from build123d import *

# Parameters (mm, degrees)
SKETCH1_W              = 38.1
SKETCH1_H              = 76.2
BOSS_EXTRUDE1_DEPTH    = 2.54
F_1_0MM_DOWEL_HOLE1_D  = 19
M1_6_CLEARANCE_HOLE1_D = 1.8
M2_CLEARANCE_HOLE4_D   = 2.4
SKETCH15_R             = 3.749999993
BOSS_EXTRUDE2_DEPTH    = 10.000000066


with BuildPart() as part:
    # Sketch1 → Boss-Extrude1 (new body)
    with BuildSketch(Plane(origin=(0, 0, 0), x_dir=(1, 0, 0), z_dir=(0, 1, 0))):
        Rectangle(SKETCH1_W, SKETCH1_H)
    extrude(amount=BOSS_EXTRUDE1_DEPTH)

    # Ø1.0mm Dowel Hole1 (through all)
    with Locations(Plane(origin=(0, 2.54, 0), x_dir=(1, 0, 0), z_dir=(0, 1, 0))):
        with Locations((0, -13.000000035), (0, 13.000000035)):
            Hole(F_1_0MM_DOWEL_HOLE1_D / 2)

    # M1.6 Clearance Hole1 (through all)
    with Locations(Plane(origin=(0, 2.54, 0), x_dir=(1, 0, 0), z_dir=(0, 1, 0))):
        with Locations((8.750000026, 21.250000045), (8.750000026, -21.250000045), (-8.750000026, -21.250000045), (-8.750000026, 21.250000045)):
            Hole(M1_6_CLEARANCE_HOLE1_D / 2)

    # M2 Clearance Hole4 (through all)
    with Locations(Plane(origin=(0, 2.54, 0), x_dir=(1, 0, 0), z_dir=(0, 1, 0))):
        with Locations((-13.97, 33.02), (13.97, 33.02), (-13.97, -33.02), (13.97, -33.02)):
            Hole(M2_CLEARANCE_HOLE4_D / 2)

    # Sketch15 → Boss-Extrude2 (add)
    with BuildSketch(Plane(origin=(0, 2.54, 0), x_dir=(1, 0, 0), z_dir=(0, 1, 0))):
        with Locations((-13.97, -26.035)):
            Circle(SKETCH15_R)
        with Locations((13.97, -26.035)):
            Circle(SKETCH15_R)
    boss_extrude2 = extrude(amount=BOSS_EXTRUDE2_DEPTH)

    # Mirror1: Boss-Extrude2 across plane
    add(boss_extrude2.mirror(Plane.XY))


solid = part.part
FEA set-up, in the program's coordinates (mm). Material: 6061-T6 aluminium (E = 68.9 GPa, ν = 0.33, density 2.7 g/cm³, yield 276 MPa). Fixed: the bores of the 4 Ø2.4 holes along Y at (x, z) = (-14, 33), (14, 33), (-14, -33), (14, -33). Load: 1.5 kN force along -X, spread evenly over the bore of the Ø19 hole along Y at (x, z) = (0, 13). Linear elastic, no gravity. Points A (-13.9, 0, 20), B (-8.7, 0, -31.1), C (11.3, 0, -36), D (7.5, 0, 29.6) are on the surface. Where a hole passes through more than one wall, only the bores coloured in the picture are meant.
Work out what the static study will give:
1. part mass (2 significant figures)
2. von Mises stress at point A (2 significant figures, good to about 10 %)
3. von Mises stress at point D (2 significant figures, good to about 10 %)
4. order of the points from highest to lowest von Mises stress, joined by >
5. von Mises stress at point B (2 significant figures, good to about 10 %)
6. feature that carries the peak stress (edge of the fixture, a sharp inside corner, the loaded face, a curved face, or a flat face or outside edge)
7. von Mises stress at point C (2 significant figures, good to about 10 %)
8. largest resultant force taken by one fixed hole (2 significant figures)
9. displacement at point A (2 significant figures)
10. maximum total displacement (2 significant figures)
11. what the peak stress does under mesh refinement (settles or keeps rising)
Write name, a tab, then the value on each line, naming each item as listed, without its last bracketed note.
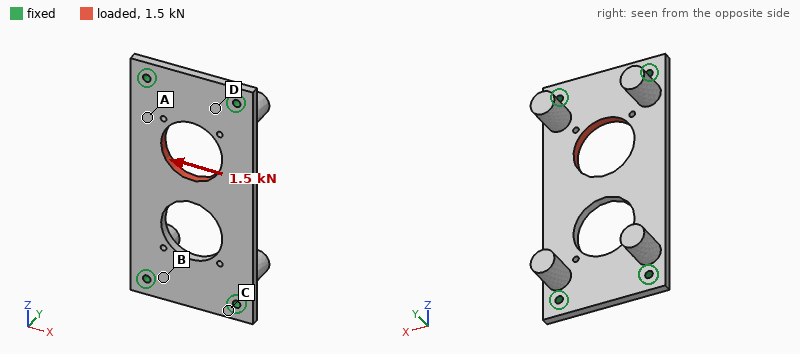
part mass	21 g
von Mises stress at point A	19 MPa
von Mises stress at point D	27 MPa
order of the points from highest to lowest von Mises stress, joined by >	D > A > B > C
von Mises stress at point B	11 MPa
feature that carries the peak stress	edge of the fixture
von Mises stress at point C	5.8 MPa
largest resultant force taken by one fixed hole	670 N
displacement at point A	11 µm
maximum total displacement	24 µm
what the peak stress does under mesh refinement	keeps rising
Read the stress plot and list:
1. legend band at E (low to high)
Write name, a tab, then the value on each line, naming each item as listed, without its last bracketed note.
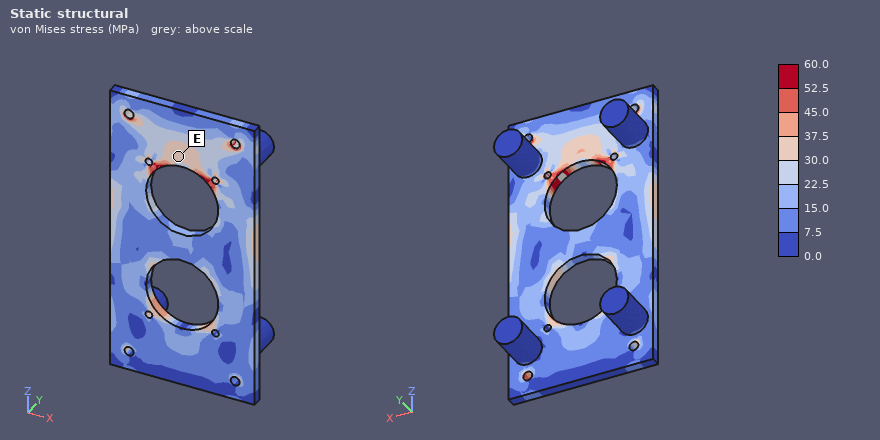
legend band at E	30.0 to 37.5 MPa
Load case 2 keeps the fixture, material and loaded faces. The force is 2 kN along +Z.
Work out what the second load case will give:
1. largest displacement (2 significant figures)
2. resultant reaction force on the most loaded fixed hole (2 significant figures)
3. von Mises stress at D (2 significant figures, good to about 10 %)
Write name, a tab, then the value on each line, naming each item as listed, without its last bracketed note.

largest displacement	12 µm
resultant reaction force on the most loaded fixed hole	710 N
von Mises stress at D	18 MPa
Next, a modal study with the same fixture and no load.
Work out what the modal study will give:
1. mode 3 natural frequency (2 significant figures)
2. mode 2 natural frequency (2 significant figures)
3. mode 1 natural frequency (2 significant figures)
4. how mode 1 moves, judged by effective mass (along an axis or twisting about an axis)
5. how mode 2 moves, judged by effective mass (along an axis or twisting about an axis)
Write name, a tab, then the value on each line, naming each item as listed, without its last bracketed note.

mode 3 natural frequency	6700 Hz
mode 2 natural frequency	4100 Hz
mode 1 natural frequency	3000 Hz
how mode 1 moves, judged by effective mass	along Y
how mode 2 moves, judged by effective mass	twisting about Z
